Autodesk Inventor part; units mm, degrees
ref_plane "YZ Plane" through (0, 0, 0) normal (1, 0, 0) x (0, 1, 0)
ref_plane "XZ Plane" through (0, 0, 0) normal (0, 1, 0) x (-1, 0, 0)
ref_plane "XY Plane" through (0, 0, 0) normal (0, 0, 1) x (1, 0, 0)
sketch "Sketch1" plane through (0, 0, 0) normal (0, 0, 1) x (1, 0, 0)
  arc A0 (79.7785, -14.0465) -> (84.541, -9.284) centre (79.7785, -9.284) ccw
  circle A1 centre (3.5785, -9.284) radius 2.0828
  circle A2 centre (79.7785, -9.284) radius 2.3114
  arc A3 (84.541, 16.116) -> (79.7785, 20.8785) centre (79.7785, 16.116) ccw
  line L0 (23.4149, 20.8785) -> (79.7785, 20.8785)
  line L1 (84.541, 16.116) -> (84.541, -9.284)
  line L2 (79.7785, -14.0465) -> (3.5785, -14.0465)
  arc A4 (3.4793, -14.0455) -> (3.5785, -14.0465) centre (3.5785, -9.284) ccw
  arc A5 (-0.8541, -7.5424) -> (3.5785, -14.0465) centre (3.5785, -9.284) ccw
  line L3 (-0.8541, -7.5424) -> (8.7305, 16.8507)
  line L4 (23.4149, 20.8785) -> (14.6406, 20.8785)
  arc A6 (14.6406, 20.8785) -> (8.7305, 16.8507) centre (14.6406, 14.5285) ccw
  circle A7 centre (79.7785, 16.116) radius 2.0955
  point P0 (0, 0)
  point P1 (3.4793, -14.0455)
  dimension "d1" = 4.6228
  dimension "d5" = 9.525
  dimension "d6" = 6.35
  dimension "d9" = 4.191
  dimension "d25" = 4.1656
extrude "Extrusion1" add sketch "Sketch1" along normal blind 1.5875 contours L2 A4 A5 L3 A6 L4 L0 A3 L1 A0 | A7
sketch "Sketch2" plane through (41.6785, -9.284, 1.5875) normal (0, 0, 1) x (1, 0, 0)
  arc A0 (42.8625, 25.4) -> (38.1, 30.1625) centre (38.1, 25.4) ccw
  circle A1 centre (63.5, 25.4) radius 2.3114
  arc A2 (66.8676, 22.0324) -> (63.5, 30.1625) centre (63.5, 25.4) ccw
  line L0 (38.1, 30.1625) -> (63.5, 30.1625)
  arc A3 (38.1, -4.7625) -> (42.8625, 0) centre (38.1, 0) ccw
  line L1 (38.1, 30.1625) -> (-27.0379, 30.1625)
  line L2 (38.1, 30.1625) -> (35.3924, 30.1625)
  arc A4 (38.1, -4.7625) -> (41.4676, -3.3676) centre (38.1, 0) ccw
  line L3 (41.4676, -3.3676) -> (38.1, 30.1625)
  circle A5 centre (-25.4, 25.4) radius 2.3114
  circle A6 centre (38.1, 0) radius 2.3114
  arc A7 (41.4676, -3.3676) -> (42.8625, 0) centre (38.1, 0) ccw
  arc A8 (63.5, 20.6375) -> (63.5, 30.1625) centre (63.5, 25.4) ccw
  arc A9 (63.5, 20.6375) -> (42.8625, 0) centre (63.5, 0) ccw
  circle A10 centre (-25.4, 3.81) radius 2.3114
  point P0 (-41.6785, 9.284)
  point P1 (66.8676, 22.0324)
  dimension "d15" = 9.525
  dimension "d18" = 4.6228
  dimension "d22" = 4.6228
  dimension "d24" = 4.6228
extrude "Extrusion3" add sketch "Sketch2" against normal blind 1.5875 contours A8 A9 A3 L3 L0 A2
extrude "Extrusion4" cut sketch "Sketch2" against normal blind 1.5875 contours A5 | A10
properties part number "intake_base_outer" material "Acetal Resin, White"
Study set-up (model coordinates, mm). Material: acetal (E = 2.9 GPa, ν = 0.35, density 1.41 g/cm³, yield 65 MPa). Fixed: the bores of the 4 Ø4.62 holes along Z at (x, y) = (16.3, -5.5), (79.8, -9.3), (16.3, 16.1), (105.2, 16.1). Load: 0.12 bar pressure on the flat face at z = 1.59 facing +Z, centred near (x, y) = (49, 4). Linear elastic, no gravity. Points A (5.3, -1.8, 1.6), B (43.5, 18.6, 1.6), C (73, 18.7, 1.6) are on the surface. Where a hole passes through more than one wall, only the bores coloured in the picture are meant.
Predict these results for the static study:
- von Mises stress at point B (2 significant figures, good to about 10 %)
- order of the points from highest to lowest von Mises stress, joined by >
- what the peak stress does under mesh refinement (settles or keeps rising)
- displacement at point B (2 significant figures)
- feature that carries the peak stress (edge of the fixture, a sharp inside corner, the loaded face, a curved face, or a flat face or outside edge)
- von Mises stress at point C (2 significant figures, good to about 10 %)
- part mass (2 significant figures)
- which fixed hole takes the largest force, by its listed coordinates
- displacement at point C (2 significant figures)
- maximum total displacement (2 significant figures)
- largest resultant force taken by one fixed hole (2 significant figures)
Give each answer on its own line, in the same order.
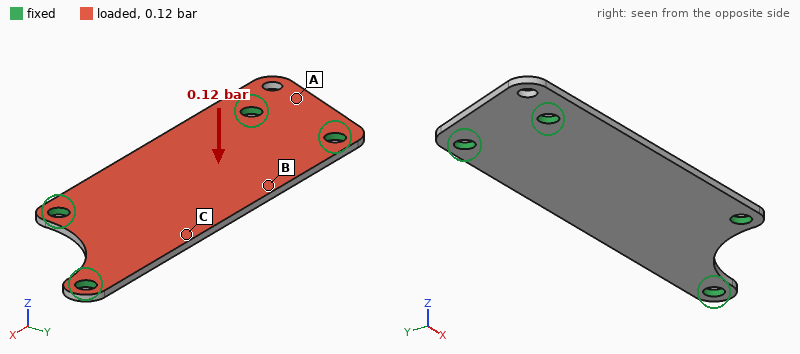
5.2 MPa
B > C > A
keeps rising
0.83 mm
edge of the fixture
2.6 MPa
6.8 g
(79.8, -9.3)
0.82 mm
1.1 mm
13 N
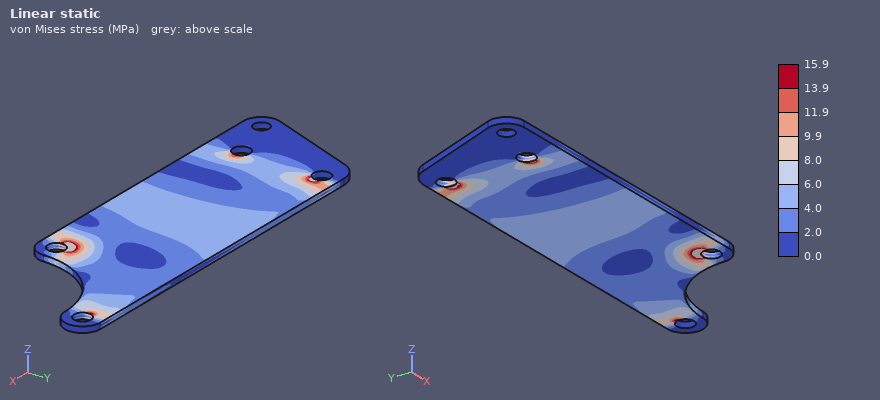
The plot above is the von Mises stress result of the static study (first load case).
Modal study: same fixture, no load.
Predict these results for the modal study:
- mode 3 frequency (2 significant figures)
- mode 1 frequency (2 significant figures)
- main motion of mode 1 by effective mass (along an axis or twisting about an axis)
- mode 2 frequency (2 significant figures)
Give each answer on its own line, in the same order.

1200 Hz
470 Hz
along Z
770 Hz
